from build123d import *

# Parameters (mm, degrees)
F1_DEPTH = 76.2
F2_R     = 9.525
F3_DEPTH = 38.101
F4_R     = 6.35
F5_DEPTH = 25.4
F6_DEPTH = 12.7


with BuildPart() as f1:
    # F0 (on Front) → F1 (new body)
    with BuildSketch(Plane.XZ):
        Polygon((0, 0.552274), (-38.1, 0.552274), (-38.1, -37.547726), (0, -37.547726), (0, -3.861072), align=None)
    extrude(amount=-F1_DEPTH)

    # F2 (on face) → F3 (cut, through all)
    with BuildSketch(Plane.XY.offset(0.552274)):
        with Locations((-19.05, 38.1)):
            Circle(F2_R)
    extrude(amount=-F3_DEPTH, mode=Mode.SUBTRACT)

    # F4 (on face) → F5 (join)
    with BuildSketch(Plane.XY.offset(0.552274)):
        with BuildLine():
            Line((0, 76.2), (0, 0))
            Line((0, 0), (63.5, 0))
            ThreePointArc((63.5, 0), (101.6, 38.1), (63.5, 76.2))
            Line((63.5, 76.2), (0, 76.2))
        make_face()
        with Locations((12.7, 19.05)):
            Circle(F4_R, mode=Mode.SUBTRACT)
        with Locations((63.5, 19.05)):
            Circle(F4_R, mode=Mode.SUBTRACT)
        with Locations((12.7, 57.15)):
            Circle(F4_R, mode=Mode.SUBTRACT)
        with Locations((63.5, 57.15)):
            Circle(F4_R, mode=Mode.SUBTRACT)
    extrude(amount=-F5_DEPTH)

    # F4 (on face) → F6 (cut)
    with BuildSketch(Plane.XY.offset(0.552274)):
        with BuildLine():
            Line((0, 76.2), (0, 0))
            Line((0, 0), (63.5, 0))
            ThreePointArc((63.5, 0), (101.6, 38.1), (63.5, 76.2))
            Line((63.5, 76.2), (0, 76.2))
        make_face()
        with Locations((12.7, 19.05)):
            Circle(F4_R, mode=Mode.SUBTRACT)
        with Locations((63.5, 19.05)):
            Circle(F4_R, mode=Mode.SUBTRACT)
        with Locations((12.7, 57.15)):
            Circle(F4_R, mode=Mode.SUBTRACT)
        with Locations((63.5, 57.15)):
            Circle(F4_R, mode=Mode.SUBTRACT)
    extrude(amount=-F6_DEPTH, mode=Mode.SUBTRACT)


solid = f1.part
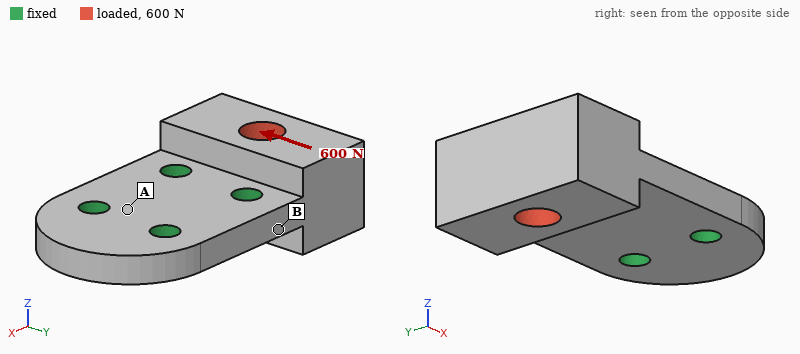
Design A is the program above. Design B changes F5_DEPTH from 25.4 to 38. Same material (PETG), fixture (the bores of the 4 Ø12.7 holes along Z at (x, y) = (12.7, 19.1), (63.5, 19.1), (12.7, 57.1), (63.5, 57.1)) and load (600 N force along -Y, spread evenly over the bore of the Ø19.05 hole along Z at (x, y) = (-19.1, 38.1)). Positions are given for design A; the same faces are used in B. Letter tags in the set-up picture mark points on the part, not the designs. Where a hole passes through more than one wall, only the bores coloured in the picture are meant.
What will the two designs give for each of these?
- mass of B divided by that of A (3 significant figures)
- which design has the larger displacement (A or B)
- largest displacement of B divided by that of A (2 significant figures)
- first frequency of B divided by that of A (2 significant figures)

1.45
A
0.70
2.2
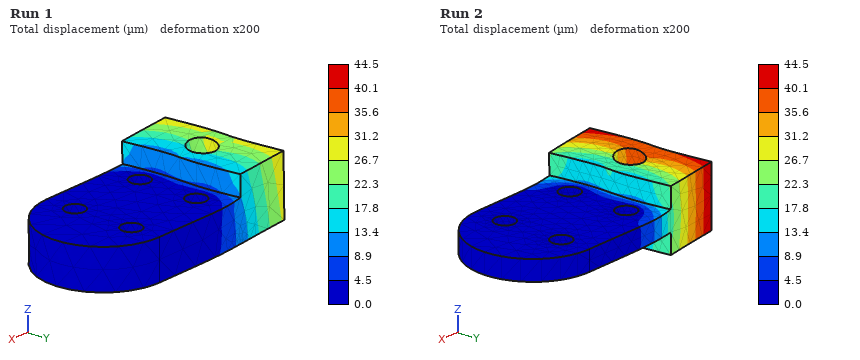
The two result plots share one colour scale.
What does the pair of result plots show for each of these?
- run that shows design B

Run 1
